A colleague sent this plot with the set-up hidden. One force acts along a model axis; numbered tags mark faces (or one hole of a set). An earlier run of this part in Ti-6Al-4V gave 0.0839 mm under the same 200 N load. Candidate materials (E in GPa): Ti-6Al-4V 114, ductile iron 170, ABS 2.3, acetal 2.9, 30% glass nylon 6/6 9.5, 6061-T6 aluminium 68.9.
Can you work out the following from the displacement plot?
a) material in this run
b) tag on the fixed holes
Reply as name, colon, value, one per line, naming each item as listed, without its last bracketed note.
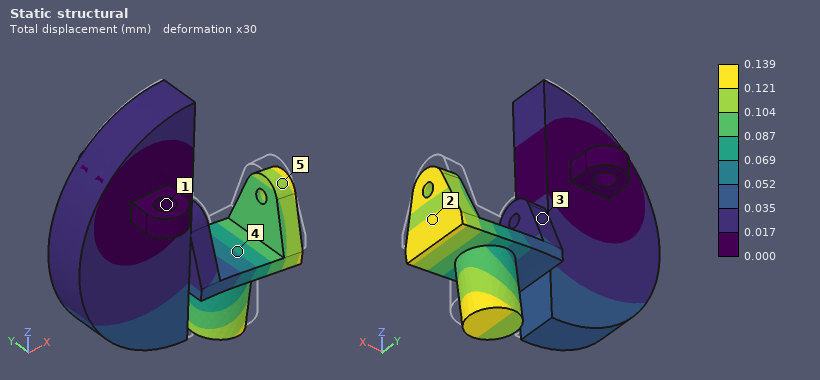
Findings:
material in this run: 6061-T6 aluminium
tag on the fixed holes: 1
